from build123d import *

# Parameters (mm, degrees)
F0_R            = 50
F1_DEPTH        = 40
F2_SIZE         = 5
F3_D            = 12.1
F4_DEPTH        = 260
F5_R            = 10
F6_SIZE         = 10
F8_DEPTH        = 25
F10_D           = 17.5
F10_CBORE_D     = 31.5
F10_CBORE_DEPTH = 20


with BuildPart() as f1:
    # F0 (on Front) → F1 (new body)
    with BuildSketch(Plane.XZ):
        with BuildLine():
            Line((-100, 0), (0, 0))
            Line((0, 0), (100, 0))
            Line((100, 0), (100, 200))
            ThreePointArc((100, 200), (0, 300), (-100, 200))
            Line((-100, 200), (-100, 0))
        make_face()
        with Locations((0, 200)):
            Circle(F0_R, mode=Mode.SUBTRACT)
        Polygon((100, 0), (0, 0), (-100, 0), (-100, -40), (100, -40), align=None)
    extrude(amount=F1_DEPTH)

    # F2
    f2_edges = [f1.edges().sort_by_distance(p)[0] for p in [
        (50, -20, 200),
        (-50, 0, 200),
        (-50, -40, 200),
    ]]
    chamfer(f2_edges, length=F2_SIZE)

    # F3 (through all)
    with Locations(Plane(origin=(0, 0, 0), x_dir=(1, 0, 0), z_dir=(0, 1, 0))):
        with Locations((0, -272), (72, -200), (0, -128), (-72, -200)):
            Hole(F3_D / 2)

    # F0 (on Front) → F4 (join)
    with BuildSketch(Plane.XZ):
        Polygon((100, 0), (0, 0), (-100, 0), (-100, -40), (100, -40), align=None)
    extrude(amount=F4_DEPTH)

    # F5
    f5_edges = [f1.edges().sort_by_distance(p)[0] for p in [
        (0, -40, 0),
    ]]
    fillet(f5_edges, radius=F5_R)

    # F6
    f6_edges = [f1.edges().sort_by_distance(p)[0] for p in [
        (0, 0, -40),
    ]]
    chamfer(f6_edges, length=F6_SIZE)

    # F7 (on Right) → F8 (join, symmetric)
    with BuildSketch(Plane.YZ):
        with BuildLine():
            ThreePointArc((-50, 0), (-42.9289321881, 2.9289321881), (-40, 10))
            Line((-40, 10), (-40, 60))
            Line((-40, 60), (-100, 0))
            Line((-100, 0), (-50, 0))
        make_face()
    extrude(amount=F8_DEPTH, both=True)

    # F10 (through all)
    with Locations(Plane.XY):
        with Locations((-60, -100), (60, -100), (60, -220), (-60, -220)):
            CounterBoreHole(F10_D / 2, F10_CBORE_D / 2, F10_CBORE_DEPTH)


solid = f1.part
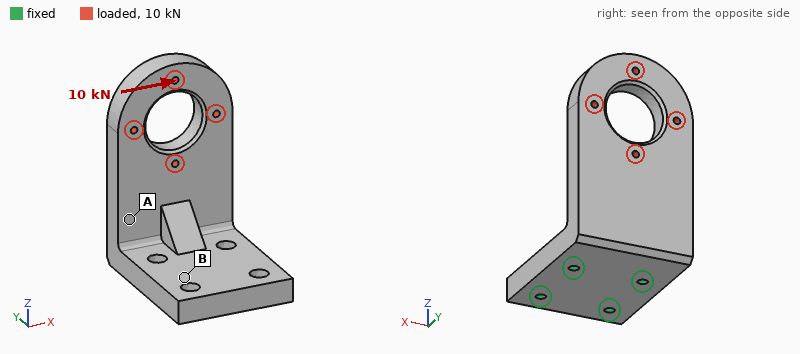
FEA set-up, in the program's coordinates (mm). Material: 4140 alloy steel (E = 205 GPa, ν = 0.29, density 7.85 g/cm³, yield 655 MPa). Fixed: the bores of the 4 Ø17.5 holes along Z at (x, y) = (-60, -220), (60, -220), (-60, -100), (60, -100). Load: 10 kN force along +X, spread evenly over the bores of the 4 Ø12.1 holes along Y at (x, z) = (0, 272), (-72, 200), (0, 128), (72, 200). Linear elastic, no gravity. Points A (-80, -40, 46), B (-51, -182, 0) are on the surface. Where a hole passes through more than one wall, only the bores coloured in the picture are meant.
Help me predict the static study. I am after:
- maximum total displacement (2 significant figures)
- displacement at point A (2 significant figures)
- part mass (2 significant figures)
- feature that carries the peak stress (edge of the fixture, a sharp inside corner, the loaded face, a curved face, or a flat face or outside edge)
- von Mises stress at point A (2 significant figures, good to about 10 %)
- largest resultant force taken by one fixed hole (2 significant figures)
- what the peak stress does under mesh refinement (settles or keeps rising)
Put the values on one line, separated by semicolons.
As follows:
93 µm; 27 µm; 31 kg; edge of the fixture; 8.3 MPa; 21 kN; keeps rising
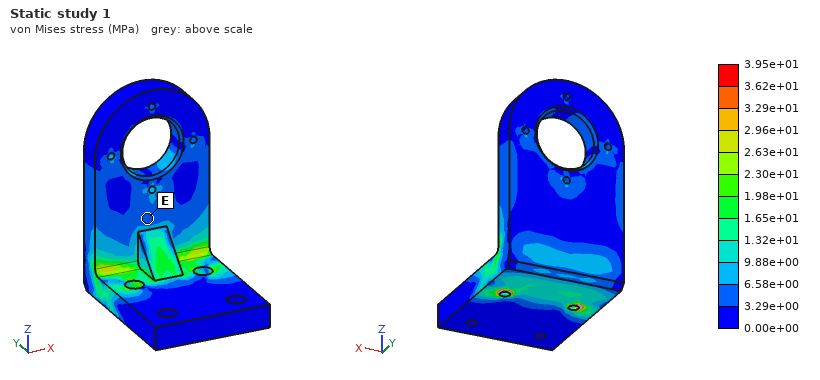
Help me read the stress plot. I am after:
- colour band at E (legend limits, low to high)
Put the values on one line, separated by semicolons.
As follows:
3.29e+00 to 6.58e+00 MPa
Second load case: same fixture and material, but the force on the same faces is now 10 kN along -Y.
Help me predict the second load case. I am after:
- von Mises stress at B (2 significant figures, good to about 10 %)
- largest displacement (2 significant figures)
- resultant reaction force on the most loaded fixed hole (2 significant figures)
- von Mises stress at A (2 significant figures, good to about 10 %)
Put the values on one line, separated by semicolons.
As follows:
6.3 MPa; 0.41 mm; 14 kN; 18 MPa
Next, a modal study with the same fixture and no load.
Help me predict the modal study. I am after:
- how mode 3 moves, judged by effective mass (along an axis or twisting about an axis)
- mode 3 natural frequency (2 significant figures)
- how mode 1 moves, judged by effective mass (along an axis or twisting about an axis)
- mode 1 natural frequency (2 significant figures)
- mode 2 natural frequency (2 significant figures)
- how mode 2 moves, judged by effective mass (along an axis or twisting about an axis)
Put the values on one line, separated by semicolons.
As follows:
along Z; 1100 Hz; along Y; 330 Hz; 640 Hz; along X
